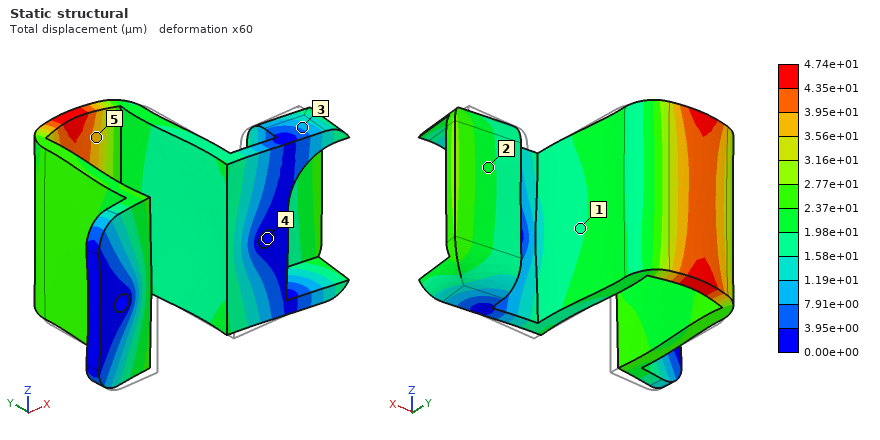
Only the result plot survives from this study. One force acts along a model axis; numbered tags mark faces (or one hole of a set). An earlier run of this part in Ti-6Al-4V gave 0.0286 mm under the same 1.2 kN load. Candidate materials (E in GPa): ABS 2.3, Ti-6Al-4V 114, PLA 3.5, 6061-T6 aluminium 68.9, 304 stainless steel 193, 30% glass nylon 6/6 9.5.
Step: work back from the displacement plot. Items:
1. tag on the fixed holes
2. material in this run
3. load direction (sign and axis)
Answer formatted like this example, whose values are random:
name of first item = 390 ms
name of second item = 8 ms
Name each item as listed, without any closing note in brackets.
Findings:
tag on the fixed holes = 4
material in this run = 6061-T6 aluminium
load direction = +Y
